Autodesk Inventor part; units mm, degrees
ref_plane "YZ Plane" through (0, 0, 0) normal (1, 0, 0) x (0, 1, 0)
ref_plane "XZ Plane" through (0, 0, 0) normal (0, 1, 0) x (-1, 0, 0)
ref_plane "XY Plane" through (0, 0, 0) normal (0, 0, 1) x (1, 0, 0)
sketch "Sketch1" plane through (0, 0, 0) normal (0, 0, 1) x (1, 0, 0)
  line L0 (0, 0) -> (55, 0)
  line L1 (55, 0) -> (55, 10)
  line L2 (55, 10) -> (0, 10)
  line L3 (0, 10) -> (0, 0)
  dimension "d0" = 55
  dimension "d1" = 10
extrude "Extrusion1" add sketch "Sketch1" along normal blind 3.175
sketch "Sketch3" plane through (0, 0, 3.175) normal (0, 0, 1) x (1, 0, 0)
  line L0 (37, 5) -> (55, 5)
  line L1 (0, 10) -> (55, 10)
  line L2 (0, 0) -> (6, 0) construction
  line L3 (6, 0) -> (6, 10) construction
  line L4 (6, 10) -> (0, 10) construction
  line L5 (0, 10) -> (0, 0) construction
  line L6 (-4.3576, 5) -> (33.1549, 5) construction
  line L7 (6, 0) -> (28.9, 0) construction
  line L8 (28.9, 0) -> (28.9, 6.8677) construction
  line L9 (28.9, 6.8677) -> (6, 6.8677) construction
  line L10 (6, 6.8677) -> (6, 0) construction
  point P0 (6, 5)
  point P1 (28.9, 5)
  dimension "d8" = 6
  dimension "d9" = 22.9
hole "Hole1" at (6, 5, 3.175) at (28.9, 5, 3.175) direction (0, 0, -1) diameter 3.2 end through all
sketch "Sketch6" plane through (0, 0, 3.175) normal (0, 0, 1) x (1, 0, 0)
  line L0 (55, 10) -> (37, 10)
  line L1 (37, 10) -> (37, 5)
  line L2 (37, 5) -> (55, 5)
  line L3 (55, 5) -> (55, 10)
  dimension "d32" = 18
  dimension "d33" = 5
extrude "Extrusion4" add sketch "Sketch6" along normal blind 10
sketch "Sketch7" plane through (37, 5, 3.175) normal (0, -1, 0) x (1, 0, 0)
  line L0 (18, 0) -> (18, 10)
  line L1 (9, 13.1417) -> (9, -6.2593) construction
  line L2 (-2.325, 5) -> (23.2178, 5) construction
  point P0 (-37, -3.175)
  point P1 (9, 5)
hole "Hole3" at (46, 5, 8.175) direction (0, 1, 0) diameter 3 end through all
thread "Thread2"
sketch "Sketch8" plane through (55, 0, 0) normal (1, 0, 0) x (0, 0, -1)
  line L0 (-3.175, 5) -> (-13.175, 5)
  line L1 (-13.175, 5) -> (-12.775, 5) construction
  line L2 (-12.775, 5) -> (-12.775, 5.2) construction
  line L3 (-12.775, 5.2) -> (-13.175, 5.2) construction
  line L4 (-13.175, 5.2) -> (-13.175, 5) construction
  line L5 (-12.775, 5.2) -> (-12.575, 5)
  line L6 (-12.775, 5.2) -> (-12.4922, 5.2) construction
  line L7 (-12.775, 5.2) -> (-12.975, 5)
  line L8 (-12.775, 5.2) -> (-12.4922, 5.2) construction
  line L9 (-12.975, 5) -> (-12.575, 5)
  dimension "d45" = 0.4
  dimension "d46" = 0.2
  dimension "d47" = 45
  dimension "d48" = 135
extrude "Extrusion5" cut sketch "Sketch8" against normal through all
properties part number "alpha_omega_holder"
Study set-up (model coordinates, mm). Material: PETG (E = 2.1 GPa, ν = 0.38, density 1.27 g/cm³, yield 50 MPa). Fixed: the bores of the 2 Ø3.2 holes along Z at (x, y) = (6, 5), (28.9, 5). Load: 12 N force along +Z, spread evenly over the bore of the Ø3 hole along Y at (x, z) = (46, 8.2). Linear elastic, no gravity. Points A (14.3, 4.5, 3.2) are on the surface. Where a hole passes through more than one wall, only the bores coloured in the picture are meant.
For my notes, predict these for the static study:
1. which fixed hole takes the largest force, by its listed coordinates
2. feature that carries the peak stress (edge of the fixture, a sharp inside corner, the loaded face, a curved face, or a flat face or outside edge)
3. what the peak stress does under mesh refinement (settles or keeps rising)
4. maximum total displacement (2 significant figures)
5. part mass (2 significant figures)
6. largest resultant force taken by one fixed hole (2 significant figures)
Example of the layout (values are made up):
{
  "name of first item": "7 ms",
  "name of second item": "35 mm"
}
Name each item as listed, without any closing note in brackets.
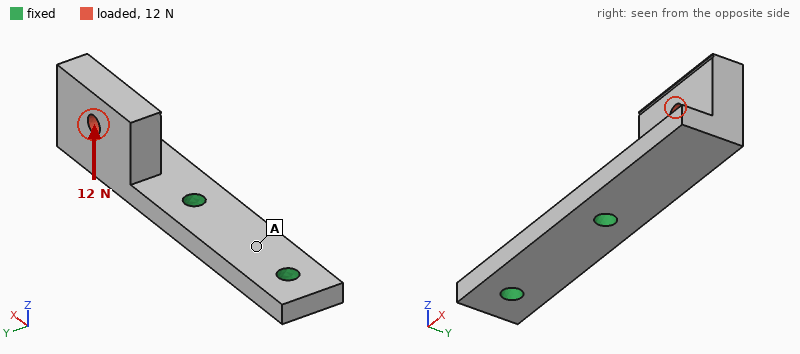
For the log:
{
  "which fixed hole takes the largest force, by its listed coordinates": "(28.9, 5)",
  "feature that carries the peak stress": "edge of the fixture",
  "what the peak stress does under mesh refinement": "keeps rising",
  "maximum total displacement": "0.60 mm",
  "part mass": "3.3 g",
  "largest resultant force taken by one fixed hole": "12 N"
}
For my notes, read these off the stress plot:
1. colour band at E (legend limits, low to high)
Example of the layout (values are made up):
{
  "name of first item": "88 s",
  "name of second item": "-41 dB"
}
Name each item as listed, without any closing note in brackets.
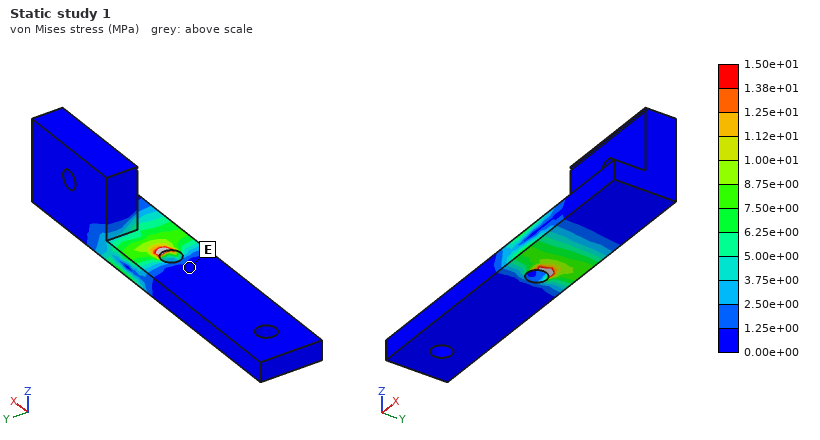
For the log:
{
  "colour band at E": "0.00e+00 to 1.25e+00 MPa"
}
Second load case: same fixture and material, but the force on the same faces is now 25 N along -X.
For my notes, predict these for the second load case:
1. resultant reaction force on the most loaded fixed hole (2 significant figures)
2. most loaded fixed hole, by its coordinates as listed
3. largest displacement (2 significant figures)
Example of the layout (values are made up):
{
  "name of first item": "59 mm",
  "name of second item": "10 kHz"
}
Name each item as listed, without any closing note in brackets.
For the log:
{
  "resultant reaction force on the most loaded fixed hole": "24 N",
  "most loaded fixed hole, by its coordinates as listed": "(28.9, 5)",
  "largest displacement": "0.68 mm"
}
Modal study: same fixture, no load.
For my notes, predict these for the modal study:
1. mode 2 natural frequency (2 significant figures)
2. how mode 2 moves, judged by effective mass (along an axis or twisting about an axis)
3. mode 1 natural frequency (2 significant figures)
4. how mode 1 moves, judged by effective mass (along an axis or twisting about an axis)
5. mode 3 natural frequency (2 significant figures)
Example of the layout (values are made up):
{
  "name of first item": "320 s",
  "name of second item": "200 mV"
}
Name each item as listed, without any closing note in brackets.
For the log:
{
  "mode 2 natural frequency": "1200 Hz",
  "how mode 2 moves, judged by effective mass": "along Y",
  "mode 1 natural frequency": "630 Hz",
  "how mode 1 moves, judged by effective mass": "along Z",
  "mode 3 natural frequency": "2400 Hz"
}
